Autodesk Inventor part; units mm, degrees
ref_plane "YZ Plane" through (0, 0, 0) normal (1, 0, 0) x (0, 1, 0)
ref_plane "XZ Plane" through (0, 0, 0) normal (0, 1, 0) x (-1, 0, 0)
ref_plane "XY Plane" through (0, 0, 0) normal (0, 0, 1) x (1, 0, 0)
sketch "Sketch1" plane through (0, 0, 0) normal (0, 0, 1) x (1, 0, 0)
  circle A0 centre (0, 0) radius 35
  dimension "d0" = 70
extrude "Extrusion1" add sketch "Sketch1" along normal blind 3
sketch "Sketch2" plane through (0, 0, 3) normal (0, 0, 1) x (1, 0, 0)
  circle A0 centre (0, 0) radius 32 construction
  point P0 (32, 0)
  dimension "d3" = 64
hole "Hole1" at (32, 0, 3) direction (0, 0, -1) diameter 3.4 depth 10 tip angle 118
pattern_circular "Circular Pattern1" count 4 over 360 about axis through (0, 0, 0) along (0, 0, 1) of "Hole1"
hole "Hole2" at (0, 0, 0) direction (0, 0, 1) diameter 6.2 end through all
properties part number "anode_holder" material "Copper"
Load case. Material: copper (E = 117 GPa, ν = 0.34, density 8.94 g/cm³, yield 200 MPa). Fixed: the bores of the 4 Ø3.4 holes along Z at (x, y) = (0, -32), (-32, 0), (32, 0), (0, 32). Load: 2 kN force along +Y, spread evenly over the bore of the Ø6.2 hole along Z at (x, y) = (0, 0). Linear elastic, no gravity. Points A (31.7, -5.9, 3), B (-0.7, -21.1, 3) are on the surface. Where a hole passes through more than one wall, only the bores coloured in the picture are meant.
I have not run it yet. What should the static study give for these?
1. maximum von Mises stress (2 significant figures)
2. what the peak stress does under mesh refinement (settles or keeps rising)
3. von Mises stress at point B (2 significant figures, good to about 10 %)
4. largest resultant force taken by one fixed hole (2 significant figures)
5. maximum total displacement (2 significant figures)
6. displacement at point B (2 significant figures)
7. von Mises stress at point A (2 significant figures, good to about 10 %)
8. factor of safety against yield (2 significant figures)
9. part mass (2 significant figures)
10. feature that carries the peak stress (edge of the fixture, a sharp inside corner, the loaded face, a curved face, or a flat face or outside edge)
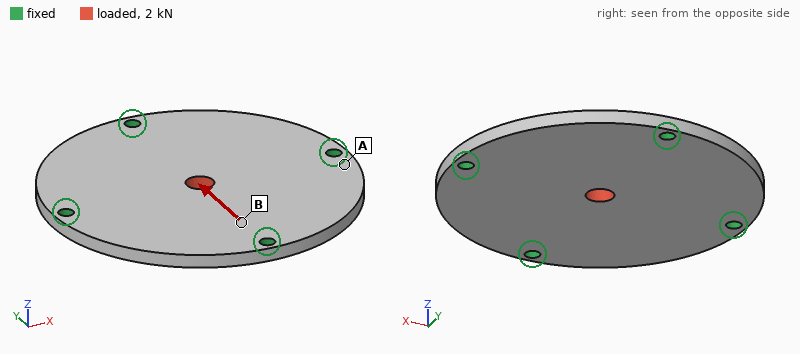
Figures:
59 MPa
settles
18 MPa
650 N
5.1 µm
1.8 µm
7.2 MPa
3.4
100 g
the loaded face
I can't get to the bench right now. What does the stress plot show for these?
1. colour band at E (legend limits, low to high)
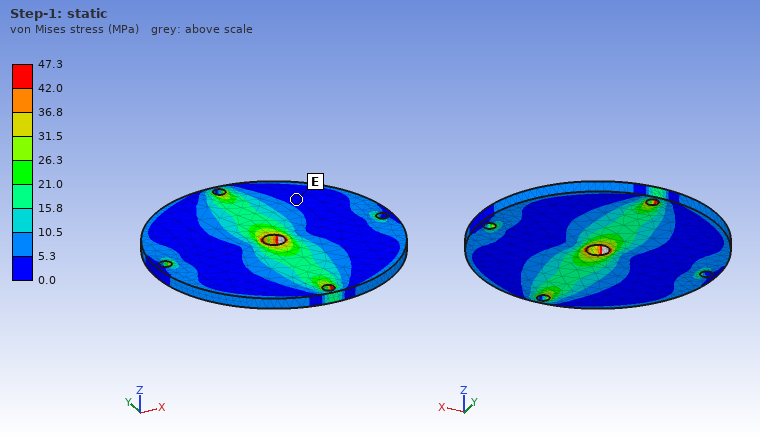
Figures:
0.0 to 5.3 MPa
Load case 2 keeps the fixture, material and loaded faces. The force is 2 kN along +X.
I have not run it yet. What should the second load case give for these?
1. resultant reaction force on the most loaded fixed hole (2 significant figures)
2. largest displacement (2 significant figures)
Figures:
650 N
5.1 µm
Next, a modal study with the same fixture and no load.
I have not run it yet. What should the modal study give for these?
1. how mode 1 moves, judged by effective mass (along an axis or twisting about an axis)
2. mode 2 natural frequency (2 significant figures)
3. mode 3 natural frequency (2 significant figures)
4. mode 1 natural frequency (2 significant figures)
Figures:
along Z
4600 Hz
4900 Hz
3800 Hz
